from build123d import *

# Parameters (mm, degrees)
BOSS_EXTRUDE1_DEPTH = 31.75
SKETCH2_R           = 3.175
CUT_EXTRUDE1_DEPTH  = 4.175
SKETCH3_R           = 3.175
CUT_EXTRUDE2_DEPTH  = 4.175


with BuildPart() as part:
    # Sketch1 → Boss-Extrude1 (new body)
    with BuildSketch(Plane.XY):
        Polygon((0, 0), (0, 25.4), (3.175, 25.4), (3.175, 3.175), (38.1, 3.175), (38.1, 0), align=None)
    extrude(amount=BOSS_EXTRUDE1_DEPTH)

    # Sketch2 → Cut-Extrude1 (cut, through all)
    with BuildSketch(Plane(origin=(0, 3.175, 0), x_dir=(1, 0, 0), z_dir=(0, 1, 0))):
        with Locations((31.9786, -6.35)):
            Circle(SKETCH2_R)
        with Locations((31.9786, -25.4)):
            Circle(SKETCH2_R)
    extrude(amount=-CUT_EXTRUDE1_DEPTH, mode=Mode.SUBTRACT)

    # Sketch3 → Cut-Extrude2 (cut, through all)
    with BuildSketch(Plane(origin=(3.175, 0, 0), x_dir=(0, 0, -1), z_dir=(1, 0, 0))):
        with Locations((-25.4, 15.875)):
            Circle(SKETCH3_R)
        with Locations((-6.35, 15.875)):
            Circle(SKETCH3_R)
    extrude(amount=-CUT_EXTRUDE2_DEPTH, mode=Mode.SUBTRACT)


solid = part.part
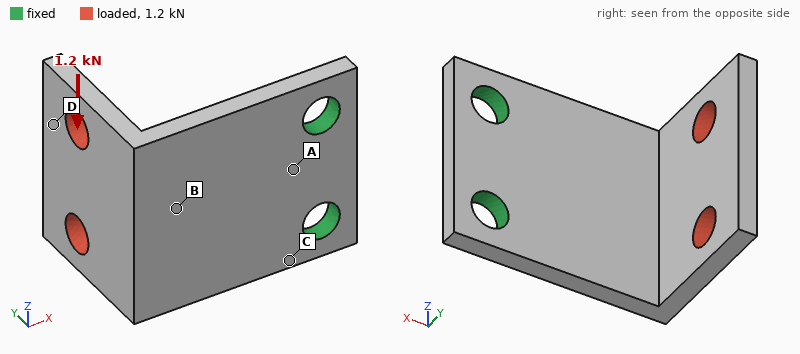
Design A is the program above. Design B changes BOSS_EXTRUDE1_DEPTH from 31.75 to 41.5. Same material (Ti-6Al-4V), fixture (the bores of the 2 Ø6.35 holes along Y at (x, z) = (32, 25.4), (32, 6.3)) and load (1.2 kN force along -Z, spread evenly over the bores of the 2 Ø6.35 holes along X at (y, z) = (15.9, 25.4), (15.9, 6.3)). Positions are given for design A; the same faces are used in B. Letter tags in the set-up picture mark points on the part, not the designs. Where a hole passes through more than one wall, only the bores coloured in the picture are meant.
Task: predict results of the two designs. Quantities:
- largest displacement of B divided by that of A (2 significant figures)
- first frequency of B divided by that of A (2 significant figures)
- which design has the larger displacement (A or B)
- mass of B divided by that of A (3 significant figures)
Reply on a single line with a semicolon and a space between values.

0.85; 0.96; A; 1.33
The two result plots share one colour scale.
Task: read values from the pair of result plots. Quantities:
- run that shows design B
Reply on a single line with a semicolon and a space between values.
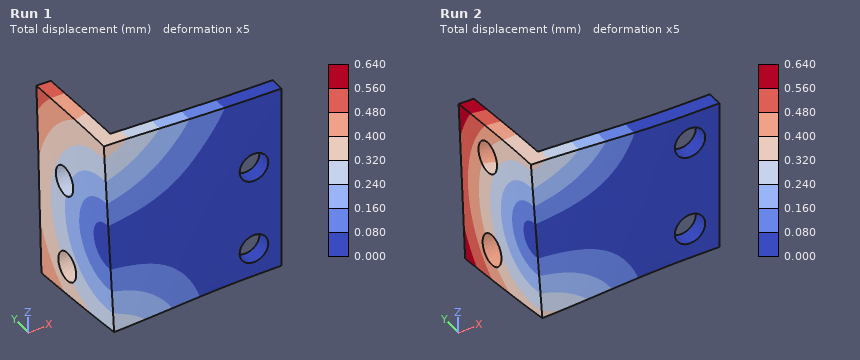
Run 1
